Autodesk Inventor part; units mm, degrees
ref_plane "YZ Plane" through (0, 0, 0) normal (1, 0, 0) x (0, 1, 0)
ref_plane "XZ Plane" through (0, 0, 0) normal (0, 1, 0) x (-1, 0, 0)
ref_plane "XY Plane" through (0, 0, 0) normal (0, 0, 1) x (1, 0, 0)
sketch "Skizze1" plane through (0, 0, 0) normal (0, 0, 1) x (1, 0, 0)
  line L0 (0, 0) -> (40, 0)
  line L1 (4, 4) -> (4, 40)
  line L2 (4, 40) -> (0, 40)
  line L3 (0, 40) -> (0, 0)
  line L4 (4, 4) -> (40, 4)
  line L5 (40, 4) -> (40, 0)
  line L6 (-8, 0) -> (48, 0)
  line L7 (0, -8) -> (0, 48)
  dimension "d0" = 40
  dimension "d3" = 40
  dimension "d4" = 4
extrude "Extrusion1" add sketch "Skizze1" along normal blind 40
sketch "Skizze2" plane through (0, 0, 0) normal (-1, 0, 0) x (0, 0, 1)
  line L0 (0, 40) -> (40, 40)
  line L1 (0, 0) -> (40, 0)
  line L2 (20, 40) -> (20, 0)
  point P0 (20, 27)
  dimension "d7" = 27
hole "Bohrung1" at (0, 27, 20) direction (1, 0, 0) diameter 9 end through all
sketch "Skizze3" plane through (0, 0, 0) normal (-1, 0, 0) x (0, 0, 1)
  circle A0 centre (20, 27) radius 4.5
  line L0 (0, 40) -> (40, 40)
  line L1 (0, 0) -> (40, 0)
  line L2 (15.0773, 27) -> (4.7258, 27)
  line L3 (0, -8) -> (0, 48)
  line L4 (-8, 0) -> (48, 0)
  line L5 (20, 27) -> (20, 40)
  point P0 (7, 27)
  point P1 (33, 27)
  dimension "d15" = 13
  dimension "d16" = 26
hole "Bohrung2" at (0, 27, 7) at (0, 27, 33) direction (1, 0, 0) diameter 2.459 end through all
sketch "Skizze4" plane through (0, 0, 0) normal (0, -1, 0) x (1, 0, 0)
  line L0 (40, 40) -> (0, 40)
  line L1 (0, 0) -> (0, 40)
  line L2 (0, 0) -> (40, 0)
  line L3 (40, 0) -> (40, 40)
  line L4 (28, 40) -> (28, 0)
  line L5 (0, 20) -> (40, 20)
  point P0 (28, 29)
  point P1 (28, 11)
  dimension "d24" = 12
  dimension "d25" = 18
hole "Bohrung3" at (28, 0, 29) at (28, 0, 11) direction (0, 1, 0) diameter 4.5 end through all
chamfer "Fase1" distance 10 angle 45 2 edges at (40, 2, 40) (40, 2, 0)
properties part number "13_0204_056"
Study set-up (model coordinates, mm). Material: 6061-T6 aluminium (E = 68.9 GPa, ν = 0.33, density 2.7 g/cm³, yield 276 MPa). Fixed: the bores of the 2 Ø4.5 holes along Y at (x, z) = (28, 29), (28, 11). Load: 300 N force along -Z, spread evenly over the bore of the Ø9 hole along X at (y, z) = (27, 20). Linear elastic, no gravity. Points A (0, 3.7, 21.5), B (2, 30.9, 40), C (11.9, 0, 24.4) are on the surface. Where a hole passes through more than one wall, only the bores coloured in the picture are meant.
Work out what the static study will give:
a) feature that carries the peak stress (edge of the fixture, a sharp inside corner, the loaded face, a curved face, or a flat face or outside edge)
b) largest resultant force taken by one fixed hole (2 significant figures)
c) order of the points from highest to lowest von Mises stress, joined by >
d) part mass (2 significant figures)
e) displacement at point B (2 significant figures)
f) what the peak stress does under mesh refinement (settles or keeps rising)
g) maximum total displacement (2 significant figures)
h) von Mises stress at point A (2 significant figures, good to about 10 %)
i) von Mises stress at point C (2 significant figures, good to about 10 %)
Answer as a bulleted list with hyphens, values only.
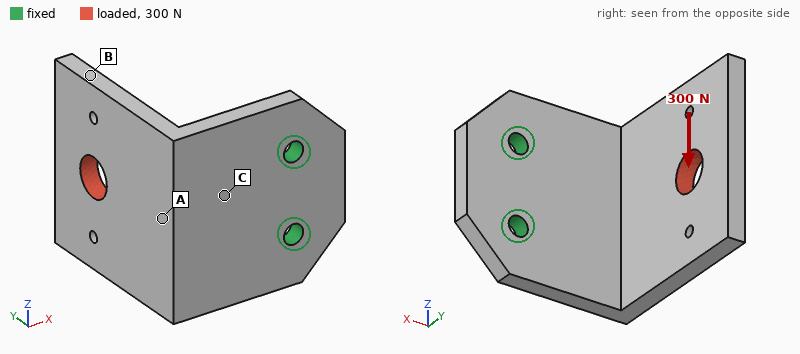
- edge of the fixture
- 490 N
- C > A > B
- 31 g
- 0.18 mm
- keeps rising
- 0.22 mm
- 25 MPa
- 37 MPa
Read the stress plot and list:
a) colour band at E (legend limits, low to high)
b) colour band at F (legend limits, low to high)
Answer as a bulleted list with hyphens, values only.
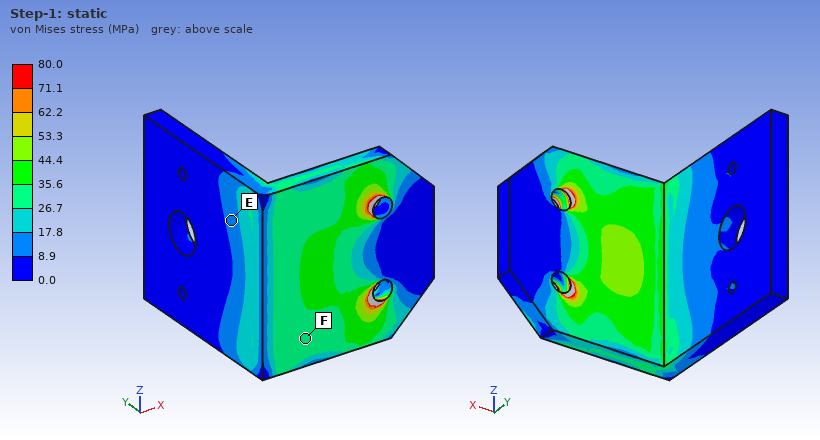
- 8.9 to 17.8 MPa
- 26.7 to 35.6 MPa
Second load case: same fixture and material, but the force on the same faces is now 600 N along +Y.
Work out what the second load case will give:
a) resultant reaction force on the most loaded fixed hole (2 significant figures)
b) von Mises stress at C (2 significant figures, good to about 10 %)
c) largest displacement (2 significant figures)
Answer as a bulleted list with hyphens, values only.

- 300 N
- 50 MPa
- 0.55 mm
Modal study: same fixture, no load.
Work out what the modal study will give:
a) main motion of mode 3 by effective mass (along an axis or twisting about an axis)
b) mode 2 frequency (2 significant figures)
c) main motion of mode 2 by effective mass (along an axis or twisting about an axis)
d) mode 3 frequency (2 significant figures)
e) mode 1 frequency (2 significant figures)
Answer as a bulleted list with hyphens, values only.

- along Y
- 1900 Hz
- along Z
- 3200 Hz
- 1100 Hz
